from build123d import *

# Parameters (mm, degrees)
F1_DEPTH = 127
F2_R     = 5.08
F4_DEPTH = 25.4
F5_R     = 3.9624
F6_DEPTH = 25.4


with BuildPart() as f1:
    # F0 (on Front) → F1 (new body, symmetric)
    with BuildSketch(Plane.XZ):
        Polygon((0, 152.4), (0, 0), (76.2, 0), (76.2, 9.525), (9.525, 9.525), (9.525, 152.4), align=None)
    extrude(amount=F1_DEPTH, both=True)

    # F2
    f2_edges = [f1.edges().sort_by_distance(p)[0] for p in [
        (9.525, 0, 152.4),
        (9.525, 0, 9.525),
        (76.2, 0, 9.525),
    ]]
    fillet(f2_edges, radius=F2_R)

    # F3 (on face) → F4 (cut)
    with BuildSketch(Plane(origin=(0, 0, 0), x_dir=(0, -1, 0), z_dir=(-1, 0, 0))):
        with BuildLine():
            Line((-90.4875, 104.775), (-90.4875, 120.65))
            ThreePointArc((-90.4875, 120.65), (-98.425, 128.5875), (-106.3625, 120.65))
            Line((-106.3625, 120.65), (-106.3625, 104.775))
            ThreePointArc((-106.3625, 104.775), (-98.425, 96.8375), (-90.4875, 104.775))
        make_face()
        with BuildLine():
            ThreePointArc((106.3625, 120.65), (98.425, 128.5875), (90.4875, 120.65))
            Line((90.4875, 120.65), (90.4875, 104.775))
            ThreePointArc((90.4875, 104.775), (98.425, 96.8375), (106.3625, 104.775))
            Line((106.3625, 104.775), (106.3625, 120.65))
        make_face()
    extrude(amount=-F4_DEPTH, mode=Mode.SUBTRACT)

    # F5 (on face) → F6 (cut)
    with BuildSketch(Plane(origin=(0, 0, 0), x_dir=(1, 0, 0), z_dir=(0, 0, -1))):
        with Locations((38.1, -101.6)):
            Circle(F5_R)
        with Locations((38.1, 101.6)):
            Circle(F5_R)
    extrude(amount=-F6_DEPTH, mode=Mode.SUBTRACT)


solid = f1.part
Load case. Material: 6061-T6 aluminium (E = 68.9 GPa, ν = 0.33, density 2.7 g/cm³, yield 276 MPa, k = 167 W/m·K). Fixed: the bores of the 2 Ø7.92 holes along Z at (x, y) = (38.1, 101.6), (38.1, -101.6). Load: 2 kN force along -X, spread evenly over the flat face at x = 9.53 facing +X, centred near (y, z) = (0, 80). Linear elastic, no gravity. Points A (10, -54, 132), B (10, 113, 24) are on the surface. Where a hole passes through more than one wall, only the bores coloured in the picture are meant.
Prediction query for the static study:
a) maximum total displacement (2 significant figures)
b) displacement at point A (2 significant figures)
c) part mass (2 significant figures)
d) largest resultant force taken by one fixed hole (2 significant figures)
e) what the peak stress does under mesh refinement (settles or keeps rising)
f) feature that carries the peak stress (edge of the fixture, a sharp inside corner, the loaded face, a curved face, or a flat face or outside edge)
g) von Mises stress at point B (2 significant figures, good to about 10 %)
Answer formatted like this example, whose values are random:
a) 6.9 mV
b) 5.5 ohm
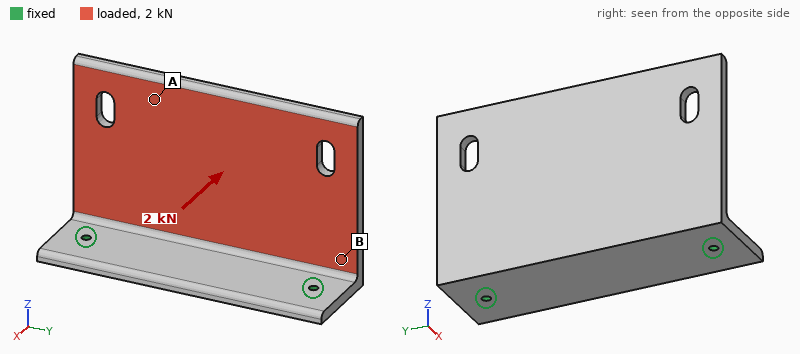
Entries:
a) 1.5 mm
b) 1.2 mm
c) 1.4 kg
d) 1.0 kN
e) keeps rising
f) edge of the fixture
g) 27 MPa
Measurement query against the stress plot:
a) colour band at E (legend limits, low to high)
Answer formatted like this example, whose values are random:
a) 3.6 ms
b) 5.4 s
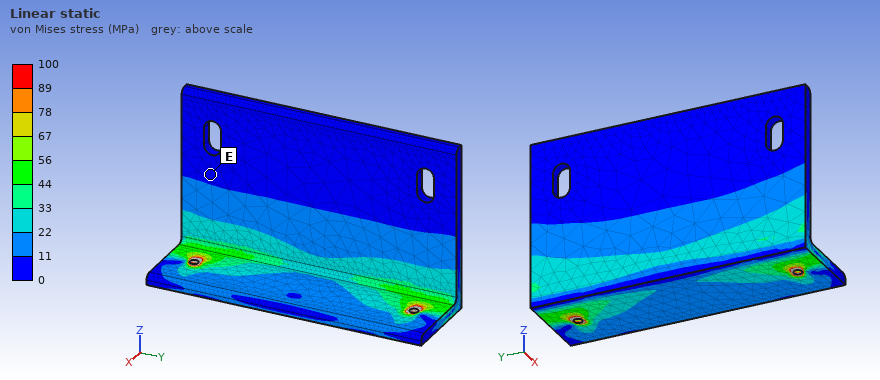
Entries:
a) 0 to 11 MPa
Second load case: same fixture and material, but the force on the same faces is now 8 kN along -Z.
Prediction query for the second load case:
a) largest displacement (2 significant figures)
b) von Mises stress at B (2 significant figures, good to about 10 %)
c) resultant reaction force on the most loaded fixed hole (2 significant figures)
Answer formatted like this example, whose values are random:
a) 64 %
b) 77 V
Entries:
a) 0.65 mm
b) 24 MPa
c) 4.0 kN
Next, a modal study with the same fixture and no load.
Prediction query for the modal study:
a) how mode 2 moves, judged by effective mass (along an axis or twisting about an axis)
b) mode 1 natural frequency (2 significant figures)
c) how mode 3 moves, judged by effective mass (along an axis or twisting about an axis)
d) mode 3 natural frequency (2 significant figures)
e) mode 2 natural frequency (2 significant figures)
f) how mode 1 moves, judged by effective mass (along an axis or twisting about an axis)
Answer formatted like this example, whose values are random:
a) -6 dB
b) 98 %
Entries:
a) twisting about Z
b) 240 Hz
c) along Z
d) 1100 Hz
e) 520 Hz
f) along X
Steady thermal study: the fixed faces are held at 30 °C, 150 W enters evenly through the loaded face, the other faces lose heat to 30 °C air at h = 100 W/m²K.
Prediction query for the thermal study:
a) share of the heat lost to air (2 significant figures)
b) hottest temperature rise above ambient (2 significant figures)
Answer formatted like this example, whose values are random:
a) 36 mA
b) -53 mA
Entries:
a) 69 %
b) 21 K
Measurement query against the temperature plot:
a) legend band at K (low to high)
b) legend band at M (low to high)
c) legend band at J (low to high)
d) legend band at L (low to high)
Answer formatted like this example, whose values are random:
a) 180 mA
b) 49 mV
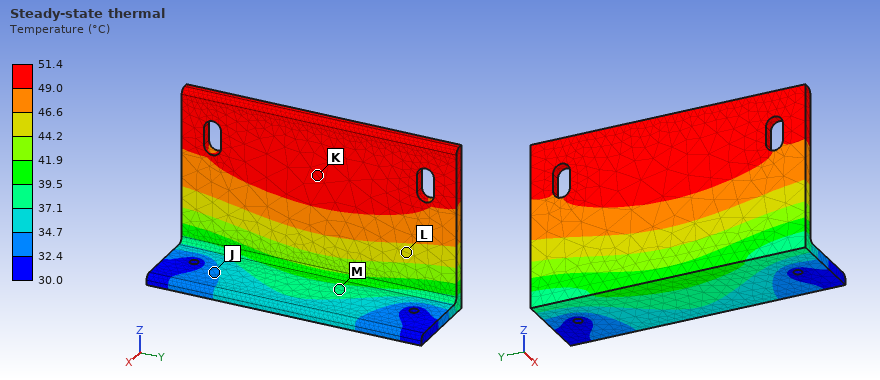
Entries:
a) 49.0 to 51.4 °C
b) 37.1 to 39.5 °C
c) 32.4 to 34.7 °C
d) 44.2 to 46.6 °C
